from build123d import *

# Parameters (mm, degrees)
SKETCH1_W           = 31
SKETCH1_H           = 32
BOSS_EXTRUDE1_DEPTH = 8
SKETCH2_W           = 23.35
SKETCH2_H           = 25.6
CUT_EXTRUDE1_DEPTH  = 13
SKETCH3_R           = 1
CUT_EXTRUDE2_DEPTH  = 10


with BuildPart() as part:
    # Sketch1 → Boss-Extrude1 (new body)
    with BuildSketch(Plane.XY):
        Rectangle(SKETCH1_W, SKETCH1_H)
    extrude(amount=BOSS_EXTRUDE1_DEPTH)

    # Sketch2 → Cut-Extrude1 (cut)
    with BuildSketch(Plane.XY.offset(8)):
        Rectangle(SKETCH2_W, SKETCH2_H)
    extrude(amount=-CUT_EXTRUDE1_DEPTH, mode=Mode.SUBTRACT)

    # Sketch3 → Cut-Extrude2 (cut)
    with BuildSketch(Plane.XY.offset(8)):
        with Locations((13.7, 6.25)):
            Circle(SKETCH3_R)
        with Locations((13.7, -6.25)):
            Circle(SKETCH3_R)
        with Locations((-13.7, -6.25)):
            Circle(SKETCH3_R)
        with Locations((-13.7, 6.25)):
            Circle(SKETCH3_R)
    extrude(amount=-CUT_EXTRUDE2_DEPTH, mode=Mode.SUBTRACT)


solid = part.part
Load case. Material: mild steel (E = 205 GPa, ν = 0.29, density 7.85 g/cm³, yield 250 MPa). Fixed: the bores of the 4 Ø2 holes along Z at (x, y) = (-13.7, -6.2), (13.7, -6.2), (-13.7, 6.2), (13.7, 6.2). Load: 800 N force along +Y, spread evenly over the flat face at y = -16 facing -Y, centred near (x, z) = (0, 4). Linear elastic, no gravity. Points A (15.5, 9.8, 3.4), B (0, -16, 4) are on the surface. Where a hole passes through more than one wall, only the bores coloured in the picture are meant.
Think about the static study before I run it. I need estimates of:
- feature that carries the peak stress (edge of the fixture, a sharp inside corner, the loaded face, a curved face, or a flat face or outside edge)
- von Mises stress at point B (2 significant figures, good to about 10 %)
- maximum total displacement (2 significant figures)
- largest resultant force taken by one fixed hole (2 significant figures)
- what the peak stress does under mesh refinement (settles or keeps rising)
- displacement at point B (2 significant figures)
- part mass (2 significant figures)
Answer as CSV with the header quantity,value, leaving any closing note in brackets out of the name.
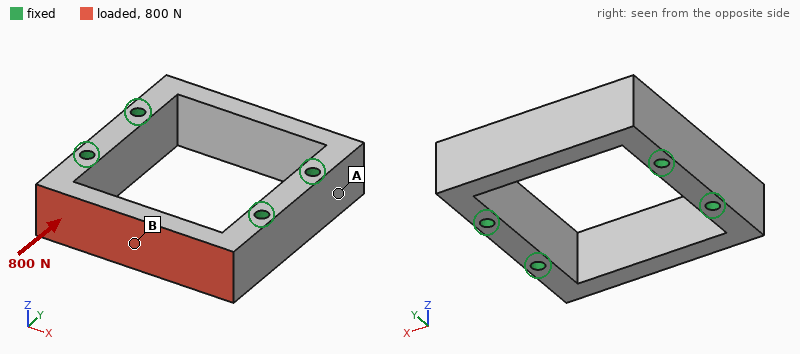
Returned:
quantity,value
feature that carries the peak stress,a sharp inside corner
von Mises stress at point B,67 MPa
maximum total displacement,11 µm
largest resultant force taken by one fixed hole,460 N
what the peak stress does under mesh refinement,keeps rising
displacement at point B,10 µm
part mass,24 g
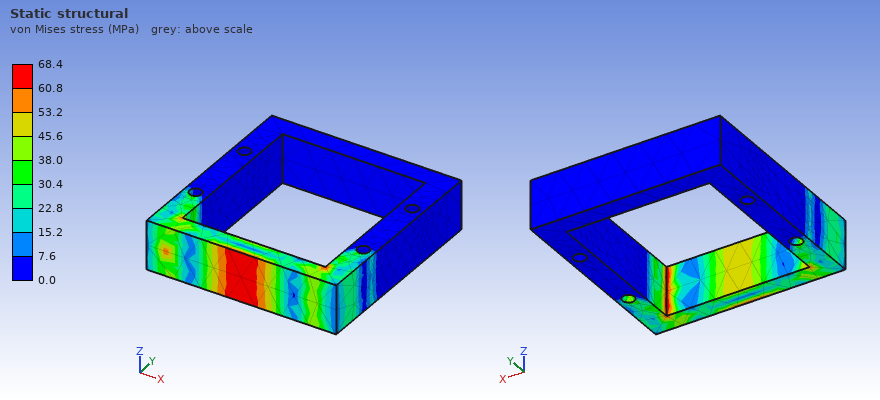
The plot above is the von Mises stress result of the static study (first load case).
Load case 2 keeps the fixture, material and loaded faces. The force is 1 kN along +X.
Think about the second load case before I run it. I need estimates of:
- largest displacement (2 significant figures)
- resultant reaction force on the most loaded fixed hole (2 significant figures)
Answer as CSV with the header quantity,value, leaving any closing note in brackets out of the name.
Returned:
quantity,value
largest displacement,10 µm
resultant reaction force on the most loaded fixed hole,550 N
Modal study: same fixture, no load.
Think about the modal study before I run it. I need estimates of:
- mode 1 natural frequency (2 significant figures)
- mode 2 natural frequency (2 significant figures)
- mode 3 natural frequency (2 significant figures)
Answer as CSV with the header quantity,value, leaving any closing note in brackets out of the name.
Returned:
quantity,value
mode 1 natural frequency,20 kHz
mode 2 natural frequency,20 kHz
mode 3 natural frequency,21 kHz
